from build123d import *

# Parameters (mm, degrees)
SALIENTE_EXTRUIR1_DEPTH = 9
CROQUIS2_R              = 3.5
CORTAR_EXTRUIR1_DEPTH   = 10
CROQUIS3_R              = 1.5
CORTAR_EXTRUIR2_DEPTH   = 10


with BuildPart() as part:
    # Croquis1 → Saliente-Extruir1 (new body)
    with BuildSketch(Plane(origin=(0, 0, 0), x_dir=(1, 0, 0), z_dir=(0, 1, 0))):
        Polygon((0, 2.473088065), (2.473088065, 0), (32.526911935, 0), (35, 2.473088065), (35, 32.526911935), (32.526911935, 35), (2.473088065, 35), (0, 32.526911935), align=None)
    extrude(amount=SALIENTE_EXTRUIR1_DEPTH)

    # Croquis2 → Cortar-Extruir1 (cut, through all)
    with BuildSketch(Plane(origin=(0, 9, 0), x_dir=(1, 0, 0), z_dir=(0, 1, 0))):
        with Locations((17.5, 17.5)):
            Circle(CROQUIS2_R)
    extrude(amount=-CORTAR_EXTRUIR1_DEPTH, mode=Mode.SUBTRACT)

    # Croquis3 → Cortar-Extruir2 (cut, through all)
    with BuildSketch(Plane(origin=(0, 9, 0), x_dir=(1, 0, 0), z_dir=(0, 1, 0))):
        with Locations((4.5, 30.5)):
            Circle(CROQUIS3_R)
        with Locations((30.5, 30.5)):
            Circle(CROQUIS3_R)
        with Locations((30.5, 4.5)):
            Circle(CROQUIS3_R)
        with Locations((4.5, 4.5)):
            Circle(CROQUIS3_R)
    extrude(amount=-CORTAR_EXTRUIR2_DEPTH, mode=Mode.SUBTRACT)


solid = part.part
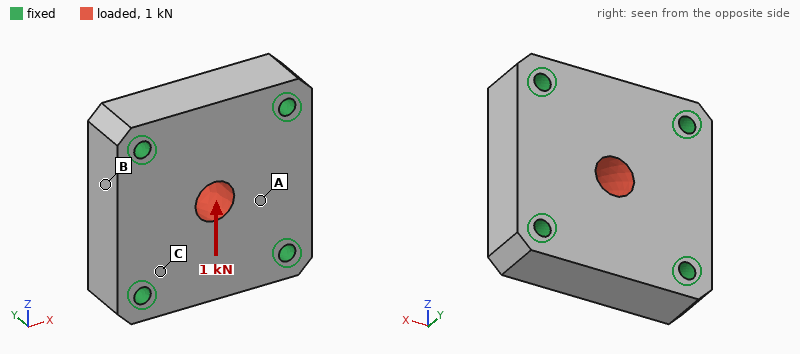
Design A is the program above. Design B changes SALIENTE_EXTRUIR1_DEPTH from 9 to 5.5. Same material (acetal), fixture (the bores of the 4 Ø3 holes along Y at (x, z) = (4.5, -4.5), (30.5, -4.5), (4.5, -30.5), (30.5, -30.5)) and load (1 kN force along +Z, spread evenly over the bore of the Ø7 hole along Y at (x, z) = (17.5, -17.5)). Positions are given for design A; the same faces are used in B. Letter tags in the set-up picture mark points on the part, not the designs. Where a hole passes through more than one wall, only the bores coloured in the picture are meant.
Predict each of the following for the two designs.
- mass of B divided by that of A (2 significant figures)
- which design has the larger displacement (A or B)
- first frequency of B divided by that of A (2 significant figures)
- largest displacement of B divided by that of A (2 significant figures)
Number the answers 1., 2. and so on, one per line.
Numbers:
1. 0.61
2. B
3. 0.77
4. 1.6
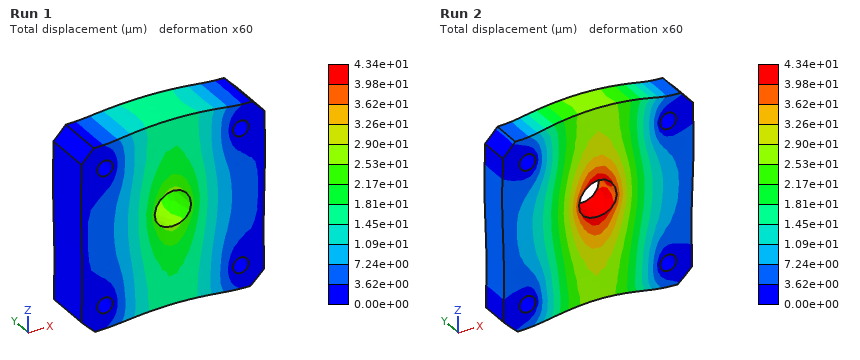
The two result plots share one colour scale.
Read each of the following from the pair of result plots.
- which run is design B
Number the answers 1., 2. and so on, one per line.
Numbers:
1. Run 2
